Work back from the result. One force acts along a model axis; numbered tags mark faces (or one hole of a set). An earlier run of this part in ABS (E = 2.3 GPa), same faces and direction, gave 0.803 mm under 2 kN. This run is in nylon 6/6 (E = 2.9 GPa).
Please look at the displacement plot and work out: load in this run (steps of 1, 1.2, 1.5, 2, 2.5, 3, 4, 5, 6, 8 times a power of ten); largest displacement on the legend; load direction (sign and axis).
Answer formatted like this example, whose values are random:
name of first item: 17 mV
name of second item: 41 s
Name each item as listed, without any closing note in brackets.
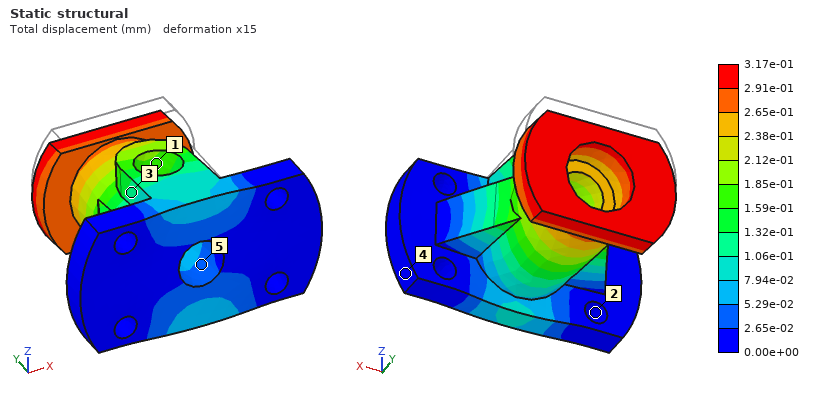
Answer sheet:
load in this run: 1 kN
largest displacement on the legend: 3.17e-01 mm
load direction: -Z
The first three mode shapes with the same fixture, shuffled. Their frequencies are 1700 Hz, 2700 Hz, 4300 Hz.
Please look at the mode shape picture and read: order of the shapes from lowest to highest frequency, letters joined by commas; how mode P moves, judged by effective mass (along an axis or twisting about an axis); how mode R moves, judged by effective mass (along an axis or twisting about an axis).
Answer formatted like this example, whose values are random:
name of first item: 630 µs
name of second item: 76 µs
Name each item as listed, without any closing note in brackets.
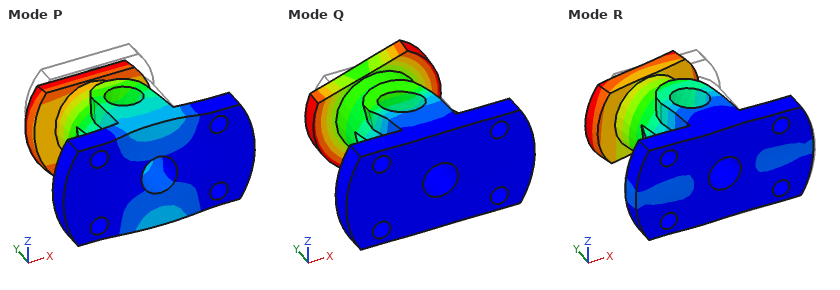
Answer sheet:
order of the shapes from lowest to highest frequency, letters joined by commas: P, R, Q
how mode P moves, judged by effective mass: along Z
how mode R moves, judged by effective mass: along X
